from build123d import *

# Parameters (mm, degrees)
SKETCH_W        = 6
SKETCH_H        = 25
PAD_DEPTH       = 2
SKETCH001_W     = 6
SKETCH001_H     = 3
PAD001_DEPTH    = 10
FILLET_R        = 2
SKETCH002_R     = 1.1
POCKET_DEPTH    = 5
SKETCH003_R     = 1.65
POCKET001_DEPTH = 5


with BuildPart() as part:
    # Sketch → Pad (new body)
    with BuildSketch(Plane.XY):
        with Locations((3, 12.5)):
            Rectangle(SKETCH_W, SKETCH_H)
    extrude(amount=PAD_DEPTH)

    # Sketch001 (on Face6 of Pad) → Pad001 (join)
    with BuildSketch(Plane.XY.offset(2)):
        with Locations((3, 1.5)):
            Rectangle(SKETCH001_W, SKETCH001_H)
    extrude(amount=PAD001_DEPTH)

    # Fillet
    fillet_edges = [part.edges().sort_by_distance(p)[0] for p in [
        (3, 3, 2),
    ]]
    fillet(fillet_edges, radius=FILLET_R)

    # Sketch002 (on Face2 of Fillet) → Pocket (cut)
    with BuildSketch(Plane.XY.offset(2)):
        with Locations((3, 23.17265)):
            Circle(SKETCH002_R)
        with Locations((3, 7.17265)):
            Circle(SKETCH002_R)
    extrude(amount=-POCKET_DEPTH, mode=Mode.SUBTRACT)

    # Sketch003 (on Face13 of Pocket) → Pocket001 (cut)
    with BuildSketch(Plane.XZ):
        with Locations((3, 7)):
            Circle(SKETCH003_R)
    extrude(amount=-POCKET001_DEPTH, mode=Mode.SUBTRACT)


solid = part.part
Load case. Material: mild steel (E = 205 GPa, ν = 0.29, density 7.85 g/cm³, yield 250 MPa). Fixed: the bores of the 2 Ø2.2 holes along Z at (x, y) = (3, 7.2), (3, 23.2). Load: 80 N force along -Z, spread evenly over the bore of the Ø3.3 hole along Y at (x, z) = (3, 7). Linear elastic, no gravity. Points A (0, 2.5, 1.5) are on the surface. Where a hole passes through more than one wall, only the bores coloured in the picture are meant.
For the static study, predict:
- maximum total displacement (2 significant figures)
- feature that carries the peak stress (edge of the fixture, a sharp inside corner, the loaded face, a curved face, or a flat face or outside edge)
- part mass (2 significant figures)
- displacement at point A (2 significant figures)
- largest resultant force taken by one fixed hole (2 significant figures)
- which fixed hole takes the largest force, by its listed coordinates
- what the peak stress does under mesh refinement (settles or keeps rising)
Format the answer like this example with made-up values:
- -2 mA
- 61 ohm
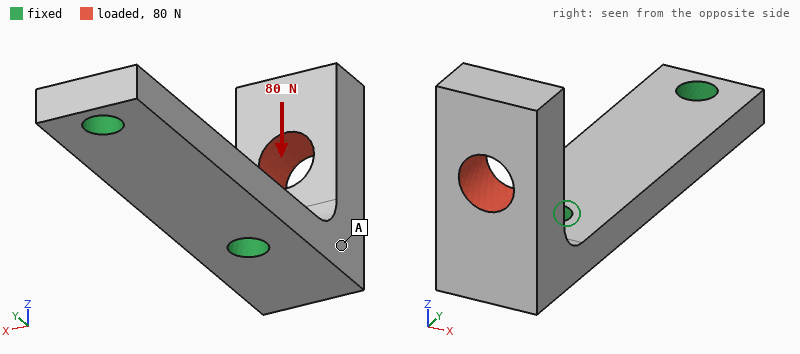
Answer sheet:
- 14 µm
- edge of the fixture
- 3.5 g
- 3.4 µm
- 81 N
- (3, 7.2)
- keeps rising
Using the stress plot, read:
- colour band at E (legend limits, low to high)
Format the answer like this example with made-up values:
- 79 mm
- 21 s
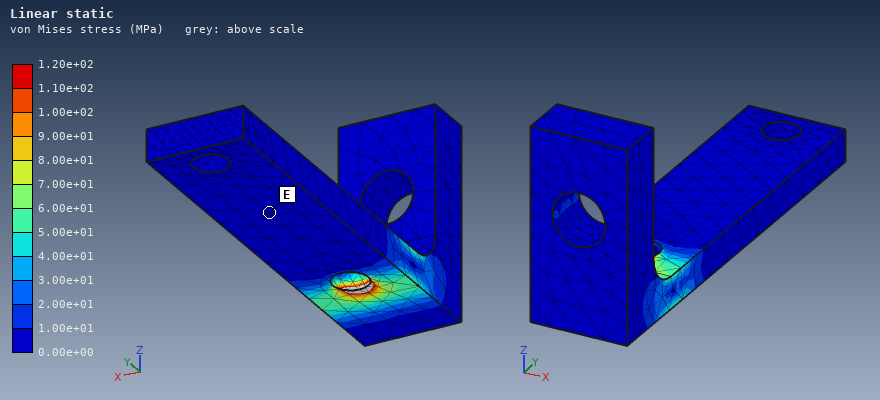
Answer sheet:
- 0.00e+00 to 1.00e+01 MPa
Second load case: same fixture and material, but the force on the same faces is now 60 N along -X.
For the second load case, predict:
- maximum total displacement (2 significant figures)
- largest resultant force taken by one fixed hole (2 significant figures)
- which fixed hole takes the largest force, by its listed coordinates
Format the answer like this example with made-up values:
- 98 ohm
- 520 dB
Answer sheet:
- 12 µm
- 67 N
- (3, 7.2)
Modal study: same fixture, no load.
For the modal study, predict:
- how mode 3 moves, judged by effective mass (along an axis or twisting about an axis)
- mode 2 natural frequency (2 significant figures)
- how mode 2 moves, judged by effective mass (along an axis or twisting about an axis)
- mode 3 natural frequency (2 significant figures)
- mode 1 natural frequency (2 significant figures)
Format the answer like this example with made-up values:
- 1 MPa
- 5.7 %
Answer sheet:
- along Z
- 12 kHz
- along X
- 32 kHz
- 8500 Hz
